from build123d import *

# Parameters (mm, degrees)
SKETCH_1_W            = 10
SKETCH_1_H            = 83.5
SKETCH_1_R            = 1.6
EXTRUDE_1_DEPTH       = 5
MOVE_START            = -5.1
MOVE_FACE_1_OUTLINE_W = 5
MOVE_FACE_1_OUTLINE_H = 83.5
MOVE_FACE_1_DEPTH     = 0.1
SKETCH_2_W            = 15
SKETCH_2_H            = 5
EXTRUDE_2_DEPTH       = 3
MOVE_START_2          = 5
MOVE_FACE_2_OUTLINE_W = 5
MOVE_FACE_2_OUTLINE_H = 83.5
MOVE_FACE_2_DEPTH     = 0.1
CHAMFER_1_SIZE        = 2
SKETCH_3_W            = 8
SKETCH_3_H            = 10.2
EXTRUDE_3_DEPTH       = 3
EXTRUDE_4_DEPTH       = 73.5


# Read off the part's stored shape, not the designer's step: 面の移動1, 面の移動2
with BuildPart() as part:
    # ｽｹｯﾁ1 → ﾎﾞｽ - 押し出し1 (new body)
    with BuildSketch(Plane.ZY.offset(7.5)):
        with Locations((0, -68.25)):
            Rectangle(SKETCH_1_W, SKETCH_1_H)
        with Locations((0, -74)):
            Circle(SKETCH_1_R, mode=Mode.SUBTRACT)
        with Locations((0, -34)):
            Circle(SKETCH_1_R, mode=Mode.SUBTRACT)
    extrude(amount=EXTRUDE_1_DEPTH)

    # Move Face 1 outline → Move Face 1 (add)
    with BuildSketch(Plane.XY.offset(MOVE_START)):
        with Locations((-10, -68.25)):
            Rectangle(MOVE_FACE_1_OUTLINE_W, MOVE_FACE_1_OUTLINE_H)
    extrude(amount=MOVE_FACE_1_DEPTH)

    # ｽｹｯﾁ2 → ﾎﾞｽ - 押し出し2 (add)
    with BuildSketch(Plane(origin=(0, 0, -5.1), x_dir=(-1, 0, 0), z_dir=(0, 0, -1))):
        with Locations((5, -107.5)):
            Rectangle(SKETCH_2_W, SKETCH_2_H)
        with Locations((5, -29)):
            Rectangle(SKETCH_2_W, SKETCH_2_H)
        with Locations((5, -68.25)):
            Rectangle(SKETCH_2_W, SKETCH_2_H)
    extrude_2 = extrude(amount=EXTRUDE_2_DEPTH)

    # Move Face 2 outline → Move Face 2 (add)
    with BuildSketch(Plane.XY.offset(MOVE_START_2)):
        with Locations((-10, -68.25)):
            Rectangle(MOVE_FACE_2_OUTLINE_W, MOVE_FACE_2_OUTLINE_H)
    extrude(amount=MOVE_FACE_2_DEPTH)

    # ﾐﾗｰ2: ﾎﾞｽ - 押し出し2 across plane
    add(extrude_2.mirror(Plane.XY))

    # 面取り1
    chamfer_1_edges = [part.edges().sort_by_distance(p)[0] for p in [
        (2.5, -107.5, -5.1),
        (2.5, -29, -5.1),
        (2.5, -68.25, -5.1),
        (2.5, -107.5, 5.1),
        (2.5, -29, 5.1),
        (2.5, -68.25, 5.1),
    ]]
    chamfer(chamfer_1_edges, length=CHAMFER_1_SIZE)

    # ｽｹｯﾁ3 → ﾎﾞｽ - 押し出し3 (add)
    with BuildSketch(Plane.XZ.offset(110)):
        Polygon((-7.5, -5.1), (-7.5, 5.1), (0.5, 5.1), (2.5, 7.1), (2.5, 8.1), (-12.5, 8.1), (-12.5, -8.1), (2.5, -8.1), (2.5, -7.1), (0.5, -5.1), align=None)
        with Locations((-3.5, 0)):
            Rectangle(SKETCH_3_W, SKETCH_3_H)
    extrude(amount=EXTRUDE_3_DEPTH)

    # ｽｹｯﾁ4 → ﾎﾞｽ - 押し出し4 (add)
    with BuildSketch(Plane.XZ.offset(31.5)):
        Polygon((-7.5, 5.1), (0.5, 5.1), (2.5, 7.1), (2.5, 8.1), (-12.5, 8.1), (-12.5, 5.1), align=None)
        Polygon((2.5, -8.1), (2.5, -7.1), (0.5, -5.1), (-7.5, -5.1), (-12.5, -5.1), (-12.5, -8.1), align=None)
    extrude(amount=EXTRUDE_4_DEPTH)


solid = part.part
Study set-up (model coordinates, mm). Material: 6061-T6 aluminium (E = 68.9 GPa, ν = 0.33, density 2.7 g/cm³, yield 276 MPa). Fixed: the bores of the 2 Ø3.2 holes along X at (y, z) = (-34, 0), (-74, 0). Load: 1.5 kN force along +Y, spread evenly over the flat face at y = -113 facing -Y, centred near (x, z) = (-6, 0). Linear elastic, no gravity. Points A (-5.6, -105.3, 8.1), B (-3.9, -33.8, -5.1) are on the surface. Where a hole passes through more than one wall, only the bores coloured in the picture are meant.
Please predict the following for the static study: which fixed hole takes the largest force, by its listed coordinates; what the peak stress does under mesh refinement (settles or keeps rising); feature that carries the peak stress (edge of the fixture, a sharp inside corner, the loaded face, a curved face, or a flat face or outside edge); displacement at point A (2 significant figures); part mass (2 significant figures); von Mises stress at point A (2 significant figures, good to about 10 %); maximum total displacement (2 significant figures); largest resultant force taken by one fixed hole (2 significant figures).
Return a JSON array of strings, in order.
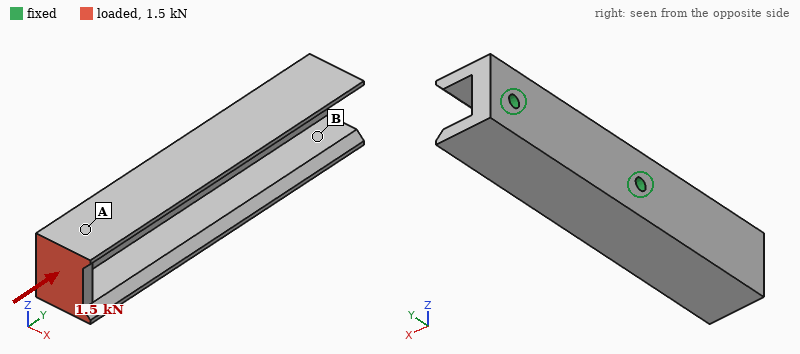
["(-74, 0)", "keeps rising", "edge of the fixture", "20 µm", "32 g", "9.1 MPa", "34 µm", "1.1 kN"]
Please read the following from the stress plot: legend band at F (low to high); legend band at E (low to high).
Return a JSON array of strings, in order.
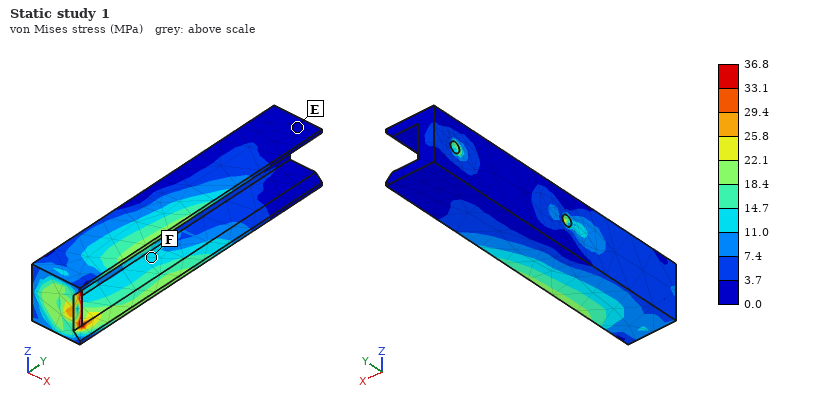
["11.0 to 14.7 MPa", "0.0 to 3.7 MPa"]
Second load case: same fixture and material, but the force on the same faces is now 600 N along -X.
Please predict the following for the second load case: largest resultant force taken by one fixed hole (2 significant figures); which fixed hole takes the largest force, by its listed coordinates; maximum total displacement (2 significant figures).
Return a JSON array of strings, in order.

["1.3 kN", "(-74, 0)", "0.15 mm"]
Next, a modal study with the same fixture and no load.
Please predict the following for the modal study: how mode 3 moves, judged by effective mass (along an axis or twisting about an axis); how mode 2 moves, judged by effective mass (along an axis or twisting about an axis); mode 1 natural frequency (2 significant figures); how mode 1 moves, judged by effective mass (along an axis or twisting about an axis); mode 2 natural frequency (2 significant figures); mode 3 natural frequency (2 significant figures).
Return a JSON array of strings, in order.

["twisting about Y", "along X", "4400 Hz", "along Z", "4600 Hz", "7900 Hz"]
